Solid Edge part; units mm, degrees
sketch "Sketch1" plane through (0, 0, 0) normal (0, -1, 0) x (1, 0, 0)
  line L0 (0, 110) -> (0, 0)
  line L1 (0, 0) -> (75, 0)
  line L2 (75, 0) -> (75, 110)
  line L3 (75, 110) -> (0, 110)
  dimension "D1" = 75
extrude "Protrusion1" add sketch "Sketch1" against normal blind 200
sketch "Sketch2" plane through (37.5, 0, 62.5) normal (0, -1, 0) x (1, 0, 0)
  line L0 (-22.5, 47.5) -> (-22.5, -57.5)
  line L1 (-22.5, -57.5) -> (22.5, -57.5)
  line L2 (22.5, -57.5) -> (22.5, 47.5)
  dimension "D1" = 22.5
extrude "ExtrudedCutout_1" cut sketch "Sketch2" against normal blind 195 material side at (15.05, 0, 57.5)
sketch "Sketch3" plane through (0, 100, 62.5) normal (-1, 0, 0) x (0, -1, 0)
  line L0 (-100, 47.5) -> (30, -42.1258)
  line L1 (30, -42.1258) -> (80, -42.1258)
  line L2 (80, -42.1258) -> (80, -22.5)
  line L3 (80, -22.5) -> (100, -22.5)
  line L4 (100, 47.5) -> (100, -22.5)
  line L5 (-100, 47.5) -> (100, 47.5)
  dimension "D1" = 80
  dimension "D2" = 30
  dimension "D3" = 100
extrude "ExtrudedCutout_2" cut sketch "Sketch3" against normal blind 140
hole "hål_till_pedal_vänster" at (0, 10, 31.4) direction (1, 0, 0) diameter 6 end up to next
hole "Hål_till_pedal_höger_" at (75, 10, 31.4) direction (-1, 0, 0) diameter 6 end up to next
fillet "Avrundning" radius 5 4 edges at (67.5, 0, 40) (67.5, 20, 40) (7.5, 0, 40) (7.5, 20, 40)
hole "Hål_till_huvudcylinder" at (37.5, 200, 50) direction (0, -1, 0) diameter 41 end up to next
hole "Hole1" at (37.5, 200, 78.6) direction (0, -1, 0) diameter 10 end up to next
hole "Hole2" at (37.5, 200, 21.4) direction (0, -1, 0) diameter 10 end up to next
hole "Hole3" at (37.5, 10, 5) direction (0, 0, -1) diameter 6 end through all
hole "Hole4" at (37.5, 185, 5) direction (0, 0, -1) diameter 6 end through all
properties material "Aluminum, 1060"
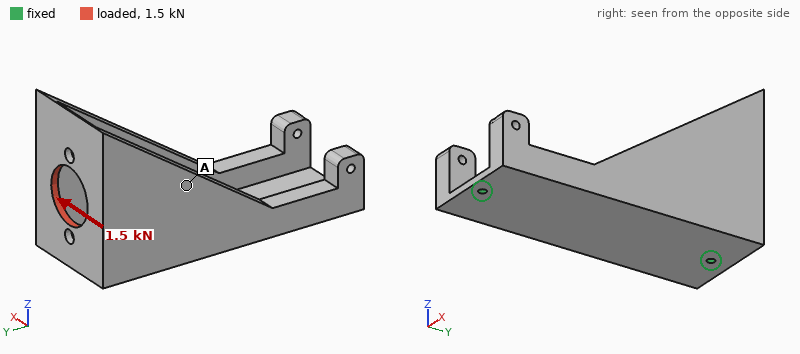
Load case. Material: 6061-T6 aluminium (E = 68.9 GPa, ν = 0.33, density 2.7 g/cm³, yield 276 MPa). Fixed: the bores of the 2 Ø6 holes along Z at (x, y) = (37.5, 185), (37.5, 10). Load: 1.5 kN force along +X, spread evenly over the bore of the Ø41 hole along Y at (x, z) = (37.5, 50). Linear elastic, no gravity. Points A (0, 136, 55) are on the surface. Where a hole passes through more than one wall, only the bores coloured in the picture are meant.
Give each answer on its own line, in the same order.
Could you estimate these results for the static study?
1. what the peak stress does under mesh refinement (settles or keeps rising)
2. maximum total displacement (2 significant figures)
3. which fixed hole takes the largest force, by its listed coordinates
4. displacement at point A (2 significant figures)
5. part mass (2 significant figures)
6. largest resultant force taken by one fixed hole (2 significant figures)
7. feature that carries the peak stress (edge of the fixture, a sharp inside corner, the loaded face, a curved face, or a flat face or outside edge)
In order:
keeps rising
0.99 mm
(37.5, 185)
0.54 mm
990 g
1.6 kN
edge of the fixture
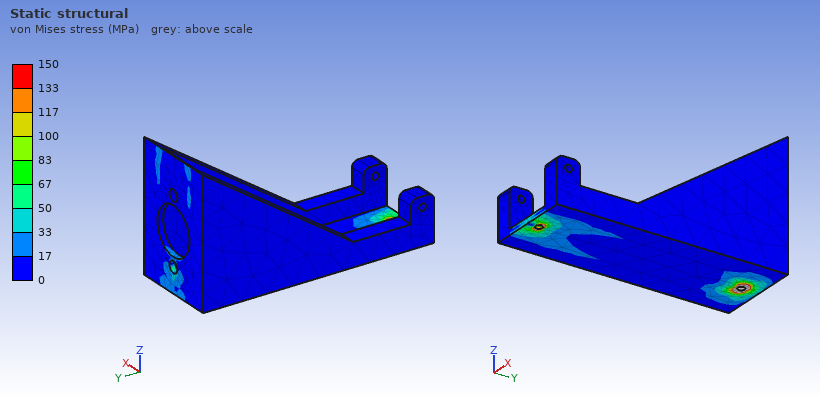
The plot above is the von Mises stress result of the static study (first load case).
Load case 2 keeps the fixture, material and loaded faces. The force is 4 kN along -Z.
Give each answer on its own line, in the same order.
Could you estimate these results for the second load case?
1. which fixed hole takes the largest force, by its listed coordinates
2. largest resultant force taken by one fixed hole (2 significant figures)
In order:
(37.5, 185)
4.2 kN
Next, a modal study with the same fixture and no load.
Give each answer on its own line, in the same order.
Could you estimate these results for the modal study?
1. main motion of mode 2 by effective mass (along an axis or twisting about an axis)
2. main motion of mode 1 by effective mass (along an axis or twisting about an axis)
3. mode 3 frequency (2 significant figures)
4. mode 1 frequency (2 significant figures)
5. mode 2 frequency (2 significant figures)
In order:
along Z
along X
1500 Hz
310 Hz
1100 Hz
